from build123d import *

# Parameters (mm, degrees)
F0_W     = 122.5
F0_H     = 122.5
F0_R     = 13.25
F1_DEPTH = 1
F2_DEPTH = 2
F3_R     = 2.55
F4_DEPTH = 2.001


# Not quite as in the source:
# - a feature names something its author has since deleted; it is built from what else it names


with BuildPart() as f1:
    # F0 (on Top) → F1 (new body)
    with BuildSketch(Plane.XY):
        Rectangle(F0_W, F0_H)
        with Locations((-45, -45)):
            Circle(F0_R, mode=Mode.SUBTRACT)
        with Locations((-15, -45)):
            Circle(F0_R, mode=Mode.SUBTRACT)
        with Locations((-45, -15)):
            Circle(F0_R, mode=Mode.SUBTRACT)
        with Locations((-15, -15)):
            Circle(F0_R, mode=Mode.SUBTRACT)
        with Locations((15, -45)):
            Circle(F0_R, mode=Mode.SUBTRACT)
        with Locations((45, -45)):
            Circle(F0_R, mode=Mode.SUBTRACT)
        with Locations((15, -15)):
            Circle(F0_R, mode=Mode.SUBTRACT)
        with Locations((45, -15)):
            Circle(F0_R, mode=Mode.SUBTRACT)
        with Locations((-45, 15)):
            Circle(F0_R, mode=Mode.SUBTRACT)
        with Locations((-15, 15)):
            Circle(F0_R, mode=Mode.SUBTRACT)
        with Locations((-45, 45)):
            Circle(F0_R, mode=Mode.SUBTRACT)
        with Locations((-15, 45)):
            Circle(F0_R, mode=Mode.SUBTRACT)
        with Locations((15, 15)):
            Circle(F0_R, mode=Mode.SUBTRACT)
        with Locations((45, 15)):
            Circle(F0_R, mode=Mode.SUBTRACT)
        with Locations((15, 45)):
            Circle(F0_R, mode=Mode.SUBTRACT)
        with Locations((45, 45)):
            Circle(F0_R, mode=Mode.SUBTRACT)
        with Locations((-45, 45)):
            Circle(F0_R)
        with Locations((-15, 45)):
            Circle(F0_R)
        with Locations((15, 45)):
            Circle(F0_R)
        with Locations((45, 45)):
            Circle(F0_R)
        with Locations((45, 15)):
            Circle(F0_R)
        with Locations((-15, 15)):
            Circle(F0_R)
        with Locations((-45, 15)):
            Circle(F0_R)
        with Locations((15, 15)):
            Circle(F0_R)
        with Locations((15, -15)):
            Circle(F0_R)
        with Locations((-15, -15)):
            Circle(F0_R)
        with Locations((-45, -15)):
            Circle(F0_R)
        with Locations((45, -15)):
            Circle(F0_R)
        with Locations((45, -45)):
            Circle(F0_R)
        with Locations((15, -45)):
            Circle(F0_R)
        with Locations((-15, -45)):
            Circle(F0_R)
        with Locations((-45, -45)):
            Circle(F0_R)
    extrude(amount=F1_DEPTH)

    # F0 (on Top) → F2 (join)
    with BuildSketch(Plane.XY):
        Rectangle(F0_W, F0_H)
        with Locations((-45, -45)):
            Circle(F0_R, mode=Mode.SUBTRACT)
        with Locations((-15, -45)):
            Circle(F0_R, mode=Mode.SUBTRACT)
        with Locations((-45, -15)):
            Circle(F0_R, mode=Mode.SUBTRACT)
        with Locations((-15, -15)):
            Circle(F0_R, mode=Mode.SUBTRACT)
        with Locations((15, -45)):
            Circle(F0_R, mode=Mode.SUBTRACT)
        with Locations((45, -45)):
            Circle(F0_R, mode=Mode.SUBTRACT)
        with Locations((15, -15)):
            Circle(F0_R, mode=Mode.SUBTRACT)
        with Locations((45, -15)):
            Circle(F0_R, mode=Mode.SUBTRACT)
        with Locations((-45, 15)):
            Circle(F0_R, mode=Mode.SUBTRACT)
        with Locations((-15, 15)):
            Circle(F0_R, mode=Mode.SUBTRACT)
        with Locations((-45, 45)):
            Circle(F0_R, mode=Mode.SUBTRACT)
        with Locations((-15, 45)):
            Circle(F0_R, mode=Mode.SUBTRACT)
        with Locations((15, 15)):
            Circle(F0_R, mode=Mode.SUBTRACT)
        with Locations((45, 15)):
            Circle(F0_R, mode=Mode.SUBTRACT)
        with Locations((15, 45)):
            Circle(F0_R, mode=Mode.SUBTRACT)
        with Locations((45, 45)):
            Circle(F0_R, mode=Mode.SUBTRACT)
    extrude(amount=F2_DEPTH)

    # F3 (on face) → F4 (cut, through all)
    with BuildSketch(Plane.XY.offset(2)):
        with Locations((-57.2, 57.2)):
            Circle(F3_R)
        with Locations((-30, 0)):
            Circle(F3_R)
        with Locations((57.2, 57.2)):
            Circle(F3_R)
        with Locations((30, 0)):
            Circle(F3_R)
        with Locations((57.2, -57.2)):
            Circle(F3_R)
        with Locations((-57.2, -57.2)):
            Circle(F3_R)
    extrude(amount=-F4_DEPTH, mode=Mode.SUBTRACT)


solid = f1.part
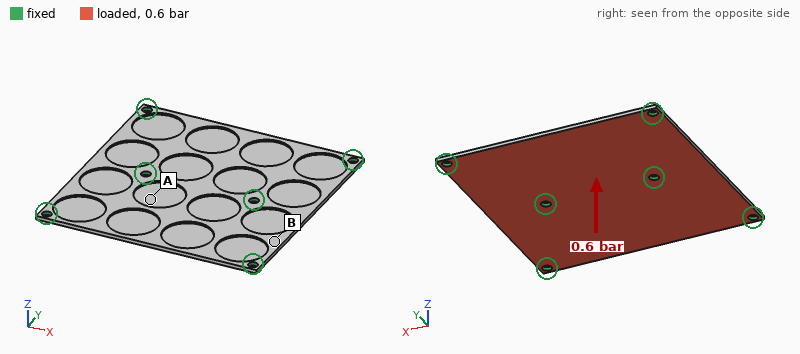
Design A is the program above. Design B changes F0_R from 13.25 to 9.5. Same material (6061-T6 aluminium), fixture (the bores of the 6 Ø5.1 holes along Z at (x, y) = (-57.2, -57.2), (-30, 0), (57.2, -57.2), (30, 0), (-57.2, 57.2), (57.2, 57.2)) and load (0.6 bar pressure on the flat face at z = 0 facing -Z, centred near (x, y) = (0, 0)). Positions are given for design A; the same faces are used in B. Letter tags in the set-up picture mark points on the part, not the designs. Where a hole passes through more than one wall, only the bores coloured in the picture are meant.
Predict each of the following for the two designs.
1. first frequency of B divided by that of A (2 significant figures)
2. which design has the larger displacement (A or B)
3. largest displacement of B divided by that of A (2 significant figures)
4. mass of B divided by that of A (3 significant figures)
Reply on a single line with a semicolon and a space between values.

1.1; A; 0.65; 1.20
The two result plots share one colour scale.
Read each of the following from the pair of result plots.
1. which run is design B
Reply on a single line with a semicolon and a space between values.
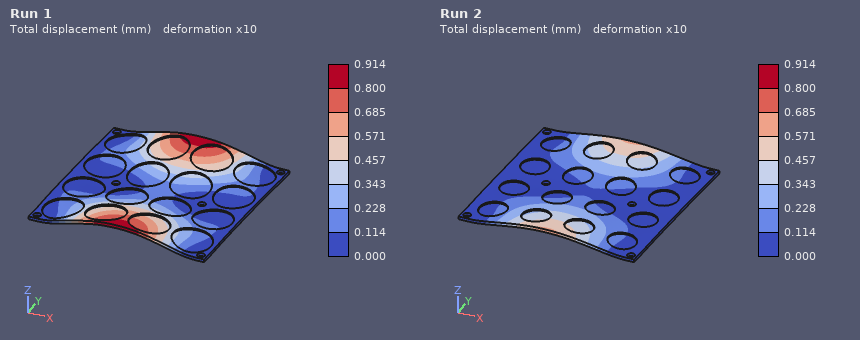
Run 2
